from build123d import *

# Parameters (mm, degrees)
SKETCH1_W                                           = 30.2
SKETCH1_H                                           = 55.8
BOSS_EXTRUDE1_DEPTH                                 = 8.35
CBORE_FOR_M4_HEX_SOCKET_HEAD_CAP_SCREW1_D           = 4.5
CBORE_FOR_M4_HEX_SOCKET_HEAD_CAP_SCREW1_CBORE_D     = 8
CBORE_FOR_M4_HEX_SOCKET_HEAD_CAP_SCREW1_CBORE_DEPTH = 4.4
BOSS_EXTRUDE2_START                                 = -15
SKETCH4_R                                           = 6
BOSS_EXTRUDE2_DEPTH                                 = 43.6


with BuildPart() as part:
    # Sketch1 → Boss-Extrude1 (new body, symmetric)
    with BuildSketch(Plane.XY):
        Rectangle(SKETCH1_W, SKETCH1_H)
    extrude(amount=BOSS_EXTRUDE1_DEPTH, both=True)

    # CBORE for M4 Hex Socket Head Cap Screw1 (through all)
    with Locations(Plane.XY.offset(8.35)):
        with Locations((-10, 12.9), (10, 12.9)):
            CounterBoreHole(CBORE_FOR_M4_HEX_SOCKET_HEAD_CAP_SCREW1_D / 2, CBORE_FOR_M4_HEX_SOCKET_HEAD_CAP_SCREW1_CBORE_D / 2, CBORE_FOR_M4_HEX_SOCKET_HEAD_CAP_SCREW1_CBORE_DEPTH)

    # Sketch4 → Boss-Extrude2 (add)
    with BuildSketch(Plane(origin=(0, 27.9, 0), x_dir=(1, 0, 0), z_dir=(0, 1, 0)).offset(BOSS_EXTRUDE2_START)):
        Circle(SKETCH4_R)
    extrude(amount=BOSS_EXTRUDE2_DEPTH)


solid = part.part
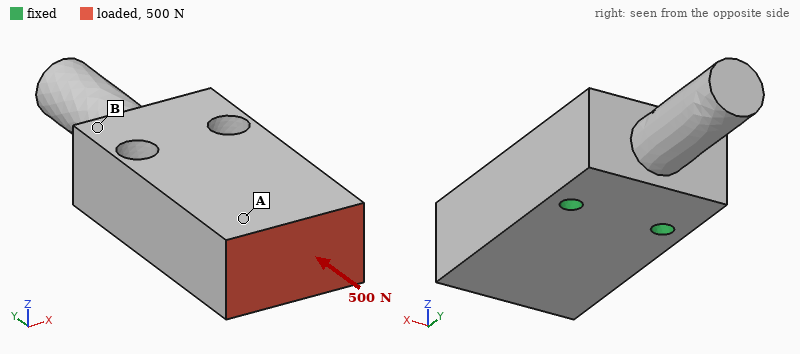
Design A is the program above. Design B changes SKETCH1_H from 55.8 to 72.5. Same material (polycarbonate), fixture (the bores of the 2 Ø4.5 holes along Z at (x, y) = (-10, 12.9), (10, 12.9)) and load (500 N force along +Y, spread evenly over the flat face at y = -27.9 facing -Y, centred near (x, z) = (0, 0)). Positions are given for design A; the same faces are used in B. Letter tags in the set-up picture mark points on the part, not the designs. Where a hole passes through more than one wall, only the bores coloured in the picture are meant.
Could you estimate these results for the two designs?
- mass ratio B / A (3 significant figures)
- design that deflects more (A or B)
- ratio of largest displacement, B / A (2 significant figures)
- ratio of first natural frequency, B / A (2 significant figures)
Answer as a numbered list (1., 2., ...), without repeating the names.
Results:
1. 1.24
2. B
3. 1.2
4. 0.75
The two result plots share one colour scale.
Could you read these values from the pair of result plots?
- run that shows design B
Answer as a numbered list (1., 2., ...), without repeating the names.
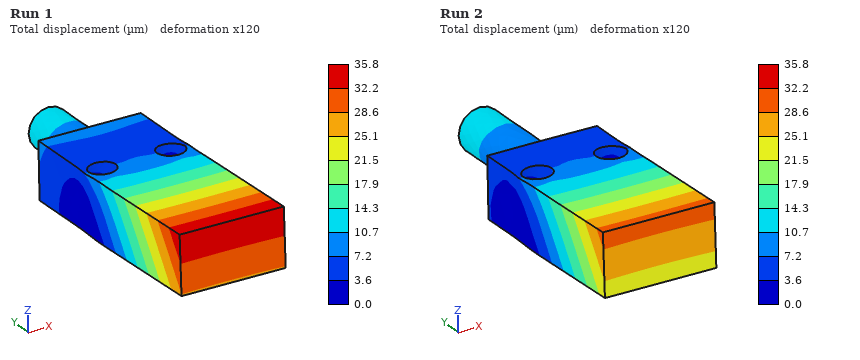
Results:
1. Run 1
